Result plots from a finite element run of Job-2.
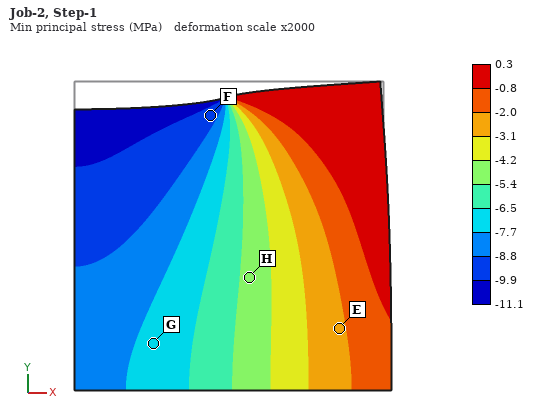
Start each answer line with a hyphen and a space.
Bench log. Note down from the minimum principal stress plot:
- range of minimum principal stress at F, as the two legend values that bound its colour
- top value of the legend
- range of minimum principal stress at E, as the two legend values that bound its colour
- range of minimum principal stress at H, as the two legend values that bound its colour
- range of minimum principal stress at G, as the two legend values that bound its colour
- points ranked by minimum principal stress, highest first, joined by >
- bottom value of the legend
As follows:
- -9.9 to -8.8 MPa
- 0.3 MPa
- -3.1 to -2.0 MPa
- -5.4 to -4.2 MPa
- -7.7 to -6.5 MPa
- E > H > G > F
- -11.1 MPa
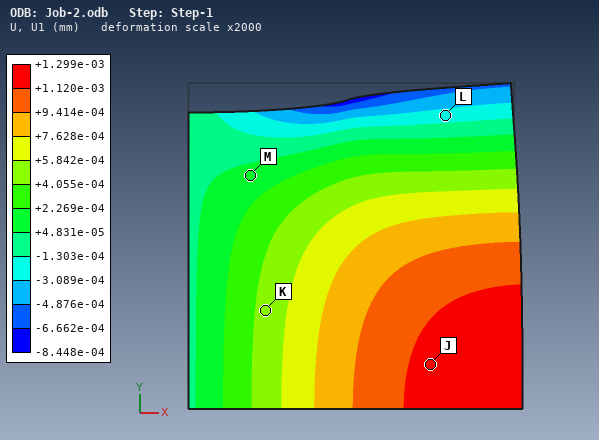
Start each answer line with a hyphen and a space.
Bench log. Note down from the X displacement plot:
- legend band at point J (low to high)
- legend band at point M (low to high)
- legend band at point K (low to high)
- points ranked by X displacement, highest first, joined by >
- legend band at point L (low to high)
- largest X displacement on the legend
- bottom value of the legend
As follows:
- +1.120e-03 to +1.299e-03 mm
- +4.831e-05 to +2.269e-04 mm
- +4.055e-04 to +5.842e-04 mm
- J > K > M > L
- -3.089e-04 to -1.303e-04 mm
- +1.299e-03 mm
- -8.448e-04 mm
